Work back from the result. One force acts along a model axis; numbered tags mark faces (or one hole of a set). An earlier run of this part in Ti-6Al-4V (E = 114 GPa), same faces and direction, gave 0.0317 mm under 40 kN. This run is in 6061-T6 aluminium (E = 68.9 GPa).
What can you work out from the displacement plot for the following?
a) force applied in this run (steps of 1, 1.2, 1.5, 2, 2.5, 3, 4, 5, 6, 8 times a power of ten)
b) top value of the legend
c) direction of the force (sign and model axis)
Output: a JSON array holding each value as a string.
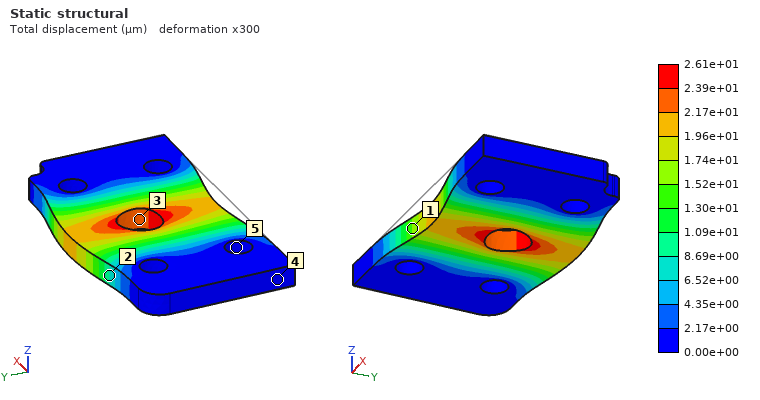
["20 kN", "2.61e+01 µm", "+Y"]
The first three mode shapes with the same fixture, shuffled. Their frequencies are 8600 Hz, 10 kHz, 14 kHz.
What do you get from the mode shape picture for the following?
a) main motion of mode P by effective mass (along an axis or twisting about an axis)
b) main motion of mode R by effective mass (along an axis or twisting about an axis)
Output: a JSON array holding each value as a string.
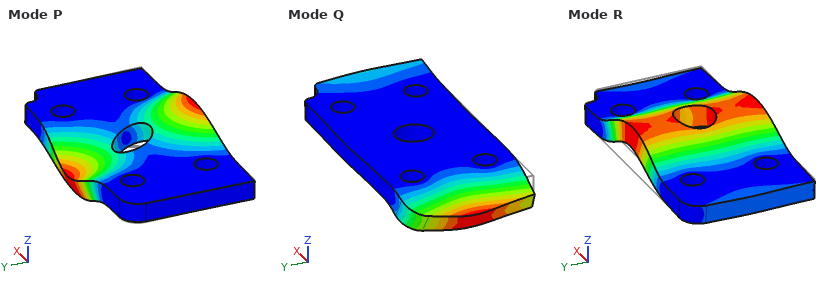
["twisting about X", "along Z"]
